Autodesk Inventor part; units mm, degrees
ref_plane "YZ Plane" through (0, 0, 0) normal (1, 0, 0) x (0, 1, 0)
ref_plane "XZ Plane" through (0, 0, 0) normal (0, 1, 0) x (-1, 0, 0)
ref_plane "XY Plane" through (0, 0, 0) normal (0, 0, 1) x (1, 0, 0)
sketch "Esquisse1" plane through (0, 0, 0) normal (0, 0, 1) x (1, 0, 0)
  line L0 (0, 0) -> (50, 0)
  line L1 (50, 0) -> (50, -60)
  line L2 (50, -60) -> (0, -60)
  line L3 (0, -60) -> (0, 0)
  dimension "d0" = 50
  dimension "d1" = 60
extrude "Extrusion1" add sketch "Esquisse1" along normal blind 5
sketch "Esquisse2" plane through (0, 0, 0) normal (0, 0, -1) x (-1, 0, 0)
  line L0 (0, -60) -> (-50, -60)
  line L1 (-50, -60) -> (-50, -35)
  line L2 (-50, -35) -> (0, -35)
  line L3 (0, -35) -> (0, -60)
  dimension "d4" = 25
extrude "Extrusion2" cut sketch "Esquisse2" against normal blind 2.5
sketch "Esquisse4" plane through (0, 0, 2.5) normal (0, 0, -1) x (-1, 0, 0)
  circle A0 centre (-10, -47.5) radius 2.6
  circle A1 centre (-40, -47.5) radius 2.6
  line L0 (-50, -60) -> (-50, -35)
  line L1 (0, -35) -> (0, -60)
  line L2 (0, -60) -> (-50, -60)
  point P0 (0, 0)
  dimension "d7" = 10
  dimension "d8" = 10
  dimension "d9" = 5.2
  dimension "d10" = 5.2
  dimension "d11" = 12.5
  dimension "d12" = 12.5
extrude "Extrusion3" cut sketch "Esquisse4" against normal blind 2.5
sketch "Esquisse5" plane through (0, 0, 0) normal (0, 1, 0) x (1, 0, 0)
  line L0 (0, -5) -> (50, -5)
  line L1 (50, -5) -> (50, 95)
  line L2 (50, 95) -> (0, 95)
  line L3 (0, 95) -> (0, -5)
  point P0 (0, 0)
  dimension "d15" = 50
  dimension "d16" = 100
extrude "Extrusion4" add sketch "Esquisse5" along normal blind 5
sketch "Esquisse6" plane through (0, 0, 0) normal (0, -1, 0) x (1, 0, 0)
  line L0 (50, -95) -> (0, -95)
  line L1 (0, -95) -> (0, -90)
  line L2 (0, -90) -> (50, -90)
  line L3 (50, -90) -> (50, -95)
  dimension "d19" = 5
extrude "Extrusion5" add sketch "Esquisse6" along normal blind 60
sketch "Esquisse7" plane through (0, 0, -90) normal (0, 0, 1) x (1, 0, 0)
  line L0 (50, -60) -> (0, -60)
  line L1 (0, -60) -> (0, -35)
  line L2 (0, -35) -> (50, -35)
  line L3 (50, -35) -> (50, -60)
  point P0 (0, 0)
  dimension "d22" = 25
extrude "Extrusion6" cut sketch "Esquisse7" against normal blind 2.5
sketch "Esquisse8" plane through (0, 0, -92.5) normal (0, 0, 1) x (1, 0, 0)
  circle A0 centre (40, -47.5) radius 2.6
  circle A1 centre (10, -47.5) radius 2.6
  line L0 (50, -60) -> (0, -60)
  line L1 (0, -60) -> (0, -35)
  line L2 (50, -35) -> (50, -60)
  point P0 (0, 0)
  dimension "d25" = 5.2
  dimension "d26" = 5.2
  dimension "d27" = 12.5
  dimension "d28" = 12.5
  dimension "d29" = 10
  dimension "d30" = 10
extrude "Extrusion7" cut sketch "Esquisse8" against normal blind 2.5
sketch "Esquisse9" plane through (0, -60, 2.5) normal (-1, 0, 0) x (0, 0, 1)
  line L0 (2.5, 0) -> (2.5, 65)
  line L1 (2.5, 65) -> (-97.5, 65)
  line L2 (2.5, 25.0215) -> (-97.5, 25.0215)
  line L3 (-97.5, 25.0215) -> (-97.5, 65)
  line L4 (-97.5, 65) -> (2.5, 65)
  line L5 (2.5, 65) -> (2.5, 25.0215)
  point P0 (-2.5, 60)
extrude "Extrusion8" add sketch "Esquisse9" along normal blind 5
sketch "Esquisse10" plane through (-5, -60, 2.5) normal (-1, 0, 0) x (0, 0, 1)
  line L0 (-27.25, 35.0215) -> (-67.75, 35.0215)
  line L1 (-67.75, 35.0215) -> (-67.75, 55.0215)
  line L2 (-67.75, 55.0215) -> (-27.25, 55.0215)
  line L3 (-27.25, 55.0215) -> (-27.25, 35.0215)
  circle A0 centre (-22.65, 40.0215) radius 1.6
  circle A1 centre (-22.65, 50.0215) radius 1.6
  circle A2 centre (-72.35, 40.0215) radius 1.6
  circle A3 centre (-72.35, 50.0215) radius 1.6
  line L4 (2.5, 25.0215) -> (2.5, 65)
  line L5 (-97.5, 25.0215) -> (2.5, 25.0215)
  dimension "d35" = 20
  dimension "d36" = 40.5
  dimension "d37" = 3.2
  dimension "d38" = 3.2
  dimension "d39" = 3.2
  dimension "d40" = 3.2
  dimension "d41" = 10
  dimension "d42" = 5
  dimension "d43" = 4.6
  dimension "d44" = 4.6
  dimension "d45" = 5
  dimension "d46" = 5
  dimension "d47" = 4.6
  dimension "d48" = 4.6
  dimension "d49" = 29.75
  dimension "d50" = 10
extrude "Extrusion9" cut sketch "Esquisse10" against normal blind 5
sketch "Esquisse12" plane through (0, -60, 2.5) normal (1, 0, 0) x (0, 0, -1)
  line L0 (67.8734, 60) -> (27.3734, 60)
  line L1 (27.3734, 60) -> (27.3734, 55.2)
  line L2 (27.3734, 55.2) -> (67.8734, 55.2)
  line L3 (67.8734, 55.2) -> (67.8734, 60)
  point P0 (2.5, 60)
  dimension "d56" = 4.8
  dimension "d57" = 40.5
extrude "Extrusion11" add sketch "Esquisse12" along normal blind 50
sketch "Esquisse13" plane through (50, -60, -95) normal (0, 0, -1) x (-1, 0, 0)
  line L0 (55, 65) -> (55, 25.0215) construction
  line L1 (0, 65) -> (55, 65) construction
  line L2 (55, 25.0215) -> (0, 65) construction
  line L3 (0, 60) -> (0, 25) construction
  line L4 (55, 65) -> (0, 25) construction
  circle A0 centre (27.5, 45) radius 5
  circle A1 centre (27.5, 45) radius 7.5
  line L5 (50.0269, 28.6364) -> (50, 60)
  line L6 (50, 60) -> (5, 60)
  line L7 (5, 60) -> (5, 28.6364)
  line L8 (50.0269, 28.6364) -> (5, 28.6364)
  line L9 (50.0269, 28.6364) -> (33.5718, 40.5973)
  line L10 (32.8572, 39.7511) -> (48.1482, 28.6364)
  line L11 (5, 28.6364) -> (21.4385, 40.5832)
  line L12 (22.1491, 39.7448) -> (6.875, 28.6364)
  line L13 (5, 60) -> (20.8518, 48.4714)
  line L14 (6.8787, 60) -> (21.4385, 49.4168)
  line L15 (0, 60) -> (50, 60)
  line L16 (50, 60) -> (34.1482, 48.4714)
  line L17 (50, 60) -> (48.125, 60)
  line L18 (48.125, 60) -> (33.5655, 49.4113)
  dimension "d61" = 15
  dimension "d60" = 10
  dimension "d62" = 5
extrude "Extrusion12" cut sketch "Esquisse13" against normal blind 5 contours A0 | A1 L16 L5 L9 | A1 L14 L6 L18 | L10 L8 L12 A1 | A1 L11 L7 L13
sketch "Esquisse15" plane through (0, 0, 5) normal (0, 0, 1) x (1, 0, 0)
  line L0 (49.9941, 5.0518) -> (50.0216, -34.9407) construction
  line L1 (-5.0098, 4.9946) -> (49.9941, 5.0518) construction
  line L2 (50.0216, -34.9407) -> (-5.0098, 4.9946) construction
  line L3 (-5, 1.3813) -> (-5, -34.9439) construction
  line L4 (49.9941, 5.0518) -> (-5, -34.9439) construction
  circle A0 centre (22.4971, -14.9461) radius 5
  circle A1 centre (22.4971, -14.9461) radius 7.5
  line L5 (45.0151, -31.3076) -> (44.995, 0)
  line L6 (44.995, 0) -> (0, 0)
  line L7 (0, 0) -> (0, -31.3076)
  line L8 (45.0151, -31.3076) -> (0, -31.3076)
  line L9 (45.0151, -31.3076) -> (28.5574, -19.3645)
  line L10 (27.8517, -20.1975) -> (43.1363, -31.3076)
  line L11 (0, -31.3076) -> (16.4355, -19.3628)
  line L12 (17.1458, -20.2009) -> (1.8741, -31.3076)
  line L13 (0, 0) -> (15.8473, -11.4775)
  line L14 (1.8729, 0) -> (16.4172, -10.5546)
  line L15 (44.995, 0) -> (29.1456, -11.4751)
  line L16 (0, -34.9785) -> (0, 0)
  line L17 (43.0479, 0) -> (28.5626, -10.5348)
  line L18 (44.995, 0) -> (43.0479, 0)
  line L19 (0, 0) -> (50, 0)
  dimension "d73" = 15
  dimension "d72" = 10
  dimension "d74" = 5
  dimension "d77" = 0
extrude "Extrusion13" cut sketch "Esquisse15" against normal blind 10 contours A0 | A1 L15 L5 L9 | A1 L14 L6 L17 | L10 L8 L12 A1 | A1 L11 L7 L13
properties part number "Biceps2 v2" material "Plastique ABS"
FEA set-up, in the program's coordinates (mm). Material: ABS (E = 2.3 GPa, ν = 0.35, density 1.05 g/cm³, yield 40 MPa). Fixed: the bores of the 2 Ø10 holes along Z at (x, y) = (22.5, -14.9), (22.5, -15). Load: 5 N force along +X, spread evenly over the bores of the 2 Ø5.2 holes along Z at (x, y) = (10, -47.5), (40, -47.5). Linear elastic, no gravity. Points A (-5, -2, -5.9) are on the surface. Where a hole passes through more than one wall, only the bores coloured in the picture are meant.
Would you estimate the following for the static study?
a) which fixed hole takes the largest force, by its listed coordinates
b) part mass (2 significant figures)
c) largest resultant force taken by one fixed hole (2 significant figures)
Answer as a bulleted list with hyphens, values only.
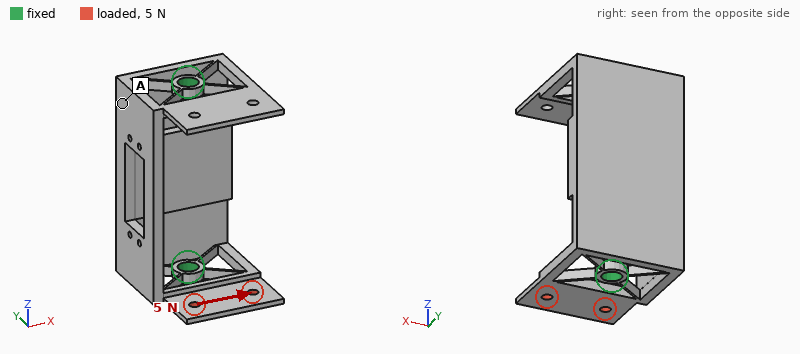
- (22.5, -15)
- 65 g
- 5.2 N
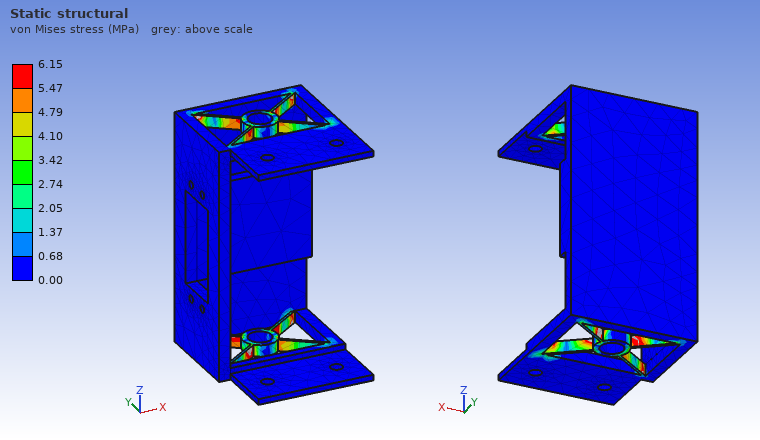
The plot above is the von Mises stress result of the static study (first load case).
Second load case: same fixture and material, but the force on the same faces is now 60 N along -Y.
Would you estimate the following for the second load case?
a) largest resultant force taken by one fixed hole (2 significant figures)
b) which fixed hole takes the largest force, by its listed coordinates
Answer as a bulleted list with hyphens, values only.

- 61 N
- (22.5, -15)
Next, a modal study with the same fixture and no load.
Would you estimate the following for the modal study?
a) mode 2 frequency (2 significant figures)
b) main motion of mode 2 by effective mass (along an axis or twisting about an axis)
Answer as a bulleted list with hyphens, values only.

- 290 Hz
- along Z
